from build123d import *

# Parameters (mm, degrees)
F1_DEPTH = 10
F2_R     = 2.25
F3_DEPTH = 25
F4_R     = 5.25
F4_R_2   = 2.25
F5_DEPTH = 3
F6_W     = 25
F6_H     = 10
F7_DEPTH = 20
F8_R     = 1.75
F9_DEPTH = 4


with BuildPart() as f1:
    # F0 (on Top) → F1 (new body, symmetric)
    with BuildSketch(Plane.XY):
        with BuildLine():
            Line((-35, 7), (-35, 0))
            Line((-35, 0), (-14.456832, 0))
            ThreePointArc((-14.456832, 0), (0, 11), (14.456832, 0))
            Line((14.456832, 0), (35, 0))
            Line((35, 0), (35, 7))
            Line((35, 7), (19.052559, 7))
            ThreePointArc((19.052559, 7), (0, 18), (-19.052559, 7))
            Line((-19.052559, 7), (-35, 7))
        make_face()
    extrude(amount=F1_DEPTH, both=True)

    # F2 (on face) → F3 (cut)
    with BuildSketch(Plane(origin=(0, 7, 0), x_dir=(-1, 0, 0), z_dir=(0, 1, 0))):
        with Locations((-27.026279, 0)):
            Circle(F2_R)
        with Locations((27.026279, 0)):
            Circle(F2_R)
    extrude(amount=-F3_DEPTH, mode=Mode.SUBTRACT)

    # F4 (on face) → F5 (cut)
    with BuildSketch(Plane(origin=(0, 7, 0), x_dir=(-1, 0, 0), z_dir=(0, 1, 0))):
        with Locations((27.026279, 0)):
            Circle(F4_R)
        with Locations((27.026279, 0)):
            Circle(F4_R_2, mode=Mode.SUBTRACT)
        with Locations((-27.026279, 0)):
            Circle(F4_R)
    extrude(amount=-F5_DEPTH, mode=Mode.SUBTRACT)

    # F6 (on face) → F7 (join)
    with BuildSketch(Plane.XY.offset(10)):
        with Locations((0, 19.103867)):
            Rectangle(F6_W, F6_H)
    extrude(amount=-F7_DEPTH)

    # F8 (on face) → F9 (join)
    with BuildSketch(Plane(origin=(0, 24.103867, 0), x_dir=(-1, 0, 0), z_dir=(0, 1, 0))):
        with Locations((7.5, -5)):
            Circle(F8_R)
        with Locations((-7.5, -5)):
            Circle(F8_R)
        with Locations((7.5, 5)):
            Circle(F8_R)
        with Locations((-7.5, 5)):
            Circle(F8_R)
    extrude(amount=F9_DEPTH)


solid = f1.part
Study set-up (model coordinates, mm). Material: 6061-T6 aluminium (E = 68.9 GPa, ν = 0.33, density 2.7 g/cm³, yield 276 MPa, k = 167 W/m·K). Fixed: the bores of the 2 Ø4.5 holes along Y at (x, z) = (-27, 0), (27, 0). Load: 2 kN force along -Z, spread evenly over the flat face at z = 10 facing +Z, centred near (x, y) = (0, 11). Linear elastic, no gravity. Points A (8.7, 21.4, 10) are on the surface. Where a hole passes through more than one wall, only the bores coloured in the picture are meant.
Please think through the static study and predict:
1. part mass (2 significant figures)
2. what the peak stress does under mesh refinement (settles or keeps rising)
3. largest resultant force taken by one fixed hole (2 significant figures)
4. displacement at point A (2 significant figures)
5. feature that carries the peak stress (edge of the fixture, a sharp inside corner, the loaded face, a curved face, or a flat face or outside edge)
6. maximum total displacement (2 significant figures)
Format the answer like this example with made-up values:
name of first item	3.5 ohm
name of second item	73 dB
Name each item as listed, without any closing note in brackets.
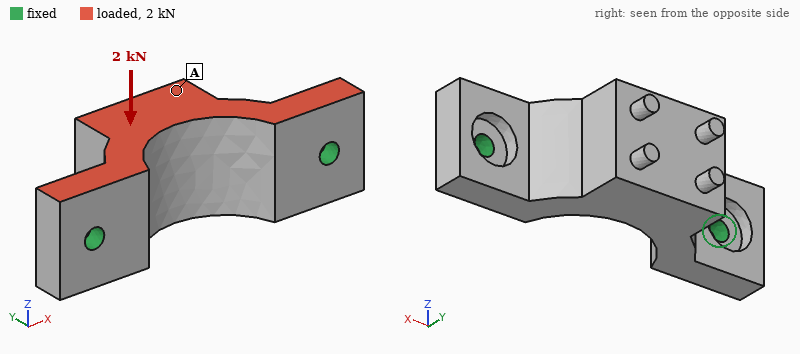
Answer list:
part mass	38 g
what the peak stress does under mesh refinement	keeps rising
largest resultant force taken by one fixed hole	1.0 kN
displacement at point A	0.096 mm
feature that carries the peak stress	edge of the fixture
maximum total displacement	0.12 mm
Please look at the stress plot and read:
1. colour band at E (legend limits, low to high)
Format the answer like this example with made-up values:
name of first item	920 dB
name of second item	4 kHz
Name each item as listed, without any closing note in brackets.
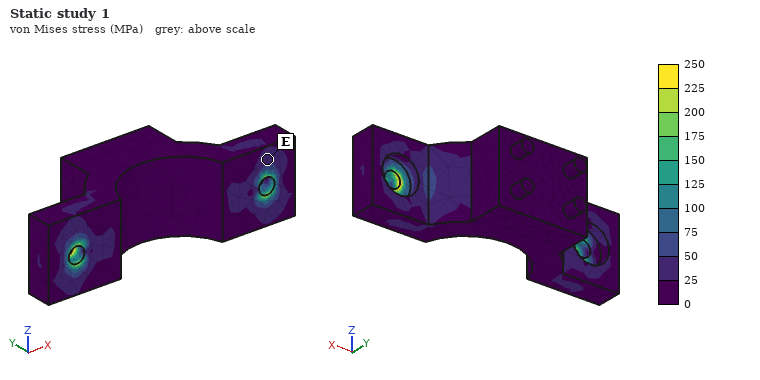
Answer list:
colour band at E	25 to 50 MPa
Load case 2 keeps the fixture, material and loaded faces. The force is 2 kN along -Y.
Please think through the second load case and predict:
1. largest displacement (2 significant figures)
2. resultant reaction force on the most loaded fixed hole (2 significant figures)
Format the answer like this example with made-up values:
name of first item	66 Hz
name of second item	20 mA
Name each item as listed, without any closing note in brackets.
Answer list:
largest displacement	0.11 mm
resultant reaction force on the most loaded fixed hole	1.2 kN
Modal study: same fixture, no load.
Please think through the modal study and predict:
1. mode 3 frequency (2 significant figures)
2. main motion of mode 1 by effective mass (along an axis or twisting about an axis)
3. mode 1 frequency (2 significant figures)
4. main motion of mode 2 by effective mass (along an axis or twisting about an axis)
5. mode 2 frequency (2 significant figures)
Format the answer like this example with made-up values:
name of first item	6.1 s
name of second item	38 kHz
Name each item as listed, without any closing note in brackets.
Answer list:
mode 3 frequency	15 kHz
main motion of mode 1 by effective mass	along Z
mode 1 frequency	4000 Hz
main motion of mode 2 by effective mass	along Y
mode 2 frequency	11 kHz
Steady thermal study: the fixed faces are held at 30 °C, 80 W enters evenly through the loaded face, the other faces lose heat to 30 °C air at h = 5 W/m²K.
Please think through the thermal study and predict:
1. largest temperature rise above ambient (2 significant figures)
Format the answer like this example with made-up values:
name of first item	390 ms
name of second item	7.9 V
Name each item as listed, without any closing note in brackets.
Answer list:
largest temperature rise above ambient	37 K
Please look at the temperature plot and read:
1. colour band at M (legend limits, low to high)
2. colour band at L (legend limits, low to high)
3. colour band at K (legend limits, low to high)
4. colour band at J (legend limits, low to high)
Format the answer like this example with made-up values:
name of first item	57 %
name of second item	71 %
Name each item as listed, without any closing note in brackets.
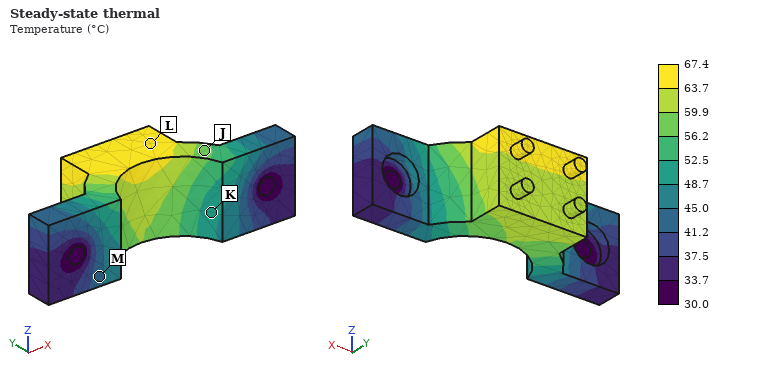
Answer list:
colour band at M	41.2 to 45.0 °C
colour band at L	63.7 to 67.4 °C
colour band at K	48.7 to 52.5 °C
colour band at J	56.2 to 59.9 °C
